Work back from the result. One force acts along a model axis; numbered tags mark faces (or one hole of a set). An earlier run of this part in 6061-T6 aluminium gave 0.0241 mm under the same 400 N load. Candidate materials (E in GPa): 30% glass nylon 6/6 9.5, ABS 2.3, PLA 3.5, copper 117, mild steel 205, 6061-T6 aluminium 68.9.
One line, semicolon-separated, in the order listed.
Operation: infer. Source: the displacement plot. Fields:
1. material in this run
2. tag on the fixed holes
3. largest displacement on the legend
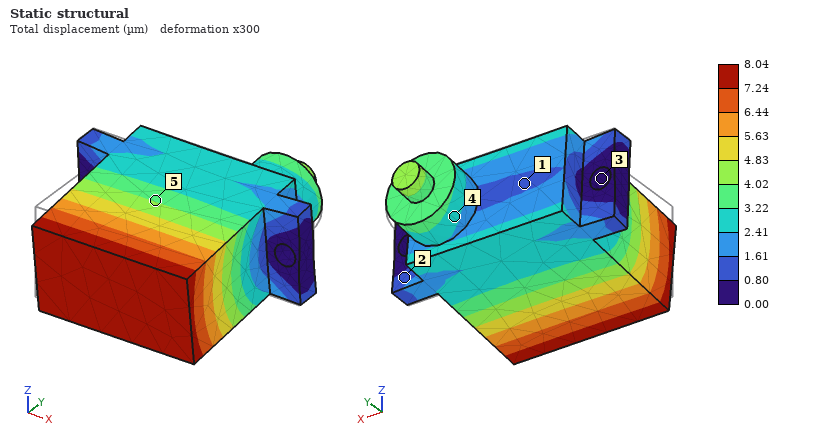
mild steel; 3; 8.04 µm
